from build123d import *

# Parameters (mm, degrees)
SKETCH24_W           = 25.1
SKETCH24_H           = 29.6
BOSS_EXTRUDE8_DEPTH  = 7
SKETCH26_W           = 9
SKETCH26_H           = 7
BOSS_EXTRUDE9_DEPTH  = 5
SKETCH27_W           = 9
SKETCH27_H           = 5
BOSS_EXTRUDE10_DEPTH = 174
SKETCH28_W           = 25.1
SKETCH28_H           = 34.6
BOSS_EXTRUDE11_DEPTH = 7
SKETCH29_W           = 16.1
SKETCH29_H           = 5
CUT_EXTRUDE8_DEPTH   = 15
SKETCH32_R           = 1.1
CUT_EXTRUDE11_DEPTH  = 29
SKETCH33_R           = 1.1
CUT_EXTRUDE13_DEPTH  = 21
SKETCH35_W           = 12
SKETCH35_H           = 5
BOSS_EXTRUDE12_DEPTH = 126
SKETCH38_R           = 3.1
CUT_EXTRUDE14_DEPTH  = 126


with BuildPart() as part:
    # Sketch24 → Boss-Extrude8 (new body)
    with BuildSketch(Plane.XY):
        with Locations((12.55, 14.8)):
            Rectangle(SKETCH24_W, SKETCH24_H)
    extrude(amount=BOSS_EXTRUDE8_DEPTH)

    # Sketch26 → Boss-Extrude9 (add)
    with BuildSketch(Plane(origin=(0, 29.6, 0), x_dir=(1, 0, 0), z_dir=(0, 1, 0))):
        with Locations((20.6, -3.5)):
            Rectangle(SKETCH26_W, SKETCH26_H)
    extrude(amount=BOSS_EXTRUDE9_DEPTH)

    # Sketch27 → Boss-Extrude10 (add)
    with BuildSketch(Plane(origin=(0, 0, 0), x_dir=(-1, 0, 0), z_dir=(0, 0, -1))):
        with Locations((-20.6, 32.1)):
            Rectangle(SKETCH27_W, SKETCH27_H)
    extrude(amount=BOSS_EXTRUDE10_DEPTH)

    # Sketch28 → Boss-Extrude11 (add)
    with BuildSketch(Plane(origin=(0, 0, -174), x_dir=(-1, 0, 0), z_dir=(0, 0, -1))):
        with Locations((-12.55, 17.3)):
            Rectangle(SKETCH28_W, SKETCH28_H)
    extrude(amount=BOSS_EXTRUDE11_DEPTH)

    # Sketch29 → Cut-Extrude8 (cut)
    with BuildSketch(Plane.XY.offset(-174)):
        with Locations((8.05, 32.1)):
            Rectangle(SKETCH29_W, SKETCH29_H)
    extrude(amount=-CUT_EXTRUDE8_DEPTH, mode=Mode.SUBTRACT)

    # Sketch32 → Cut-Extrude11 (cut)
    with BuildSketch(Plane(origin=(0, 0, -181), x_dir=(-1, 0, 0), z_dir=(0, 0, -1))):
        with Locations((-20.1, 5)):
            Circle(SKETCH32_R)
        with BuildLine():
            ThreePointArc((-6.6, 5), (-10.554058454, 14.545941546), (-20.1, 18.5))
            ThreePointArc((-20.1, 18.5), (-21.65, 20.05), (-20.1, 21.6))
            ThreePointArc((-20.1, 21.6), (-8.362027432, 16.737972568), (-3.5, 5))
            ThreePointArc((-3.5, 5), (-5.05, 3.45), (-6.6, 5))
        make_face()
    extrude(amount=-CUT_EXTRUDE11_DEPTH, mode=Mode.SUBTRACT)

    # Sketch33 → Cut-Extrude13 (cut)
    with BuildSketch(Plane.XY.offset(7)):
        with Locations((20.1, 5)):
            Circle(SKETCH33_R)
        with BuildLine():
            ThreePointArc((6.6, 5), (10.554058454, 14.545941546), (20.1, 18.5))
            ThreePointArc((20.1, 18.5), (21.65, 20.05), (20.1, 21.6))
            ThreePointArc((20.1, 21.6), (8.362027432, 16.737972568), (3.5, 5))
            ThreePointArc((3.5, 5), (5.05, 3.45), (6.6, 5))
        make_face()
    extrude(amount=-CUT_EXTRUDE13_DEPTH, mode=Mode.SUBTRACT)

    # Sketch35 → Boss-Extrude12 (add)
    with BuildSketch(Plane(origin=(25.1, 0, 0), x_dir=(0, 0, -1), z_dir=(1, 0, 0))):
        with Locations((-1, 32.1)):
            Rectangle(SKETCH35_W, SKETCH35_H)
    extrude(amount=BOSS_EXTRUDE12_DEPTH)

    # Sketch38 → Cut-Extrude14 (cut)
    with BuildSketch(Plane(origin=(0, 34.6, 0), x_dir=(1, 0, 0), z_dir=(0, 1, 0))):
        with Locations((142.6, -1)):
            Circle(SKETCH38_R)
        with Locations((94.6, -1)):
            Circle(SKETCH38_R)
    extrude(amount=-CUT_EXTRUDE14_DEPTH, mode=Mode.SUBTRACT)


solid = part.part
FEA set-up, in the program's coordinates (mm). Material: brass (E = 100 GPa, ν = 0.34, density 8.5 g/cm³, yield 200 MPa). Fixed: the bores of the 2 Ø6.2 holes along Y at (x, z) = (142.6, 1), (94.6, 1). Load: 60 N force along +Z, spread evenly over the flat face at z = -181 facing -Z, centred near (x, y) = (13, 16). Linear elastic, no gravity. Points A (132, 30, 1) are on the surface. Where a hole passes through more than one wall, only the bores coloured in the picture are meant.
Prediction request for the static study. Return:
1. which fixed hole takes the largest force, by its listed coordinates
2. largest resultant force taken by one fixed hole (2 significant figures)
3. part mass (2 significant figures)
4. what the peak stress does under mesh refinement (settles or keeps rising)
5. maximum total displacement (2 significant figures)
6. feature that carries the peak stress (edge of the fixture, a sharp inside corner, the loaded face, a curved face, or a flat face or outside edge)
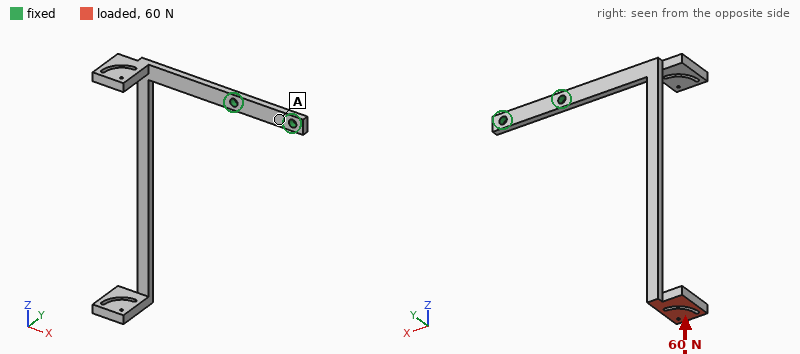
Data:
(94.6, 1)
72 N
210 g
keeps rising
2.8 mm
edge of the fixture
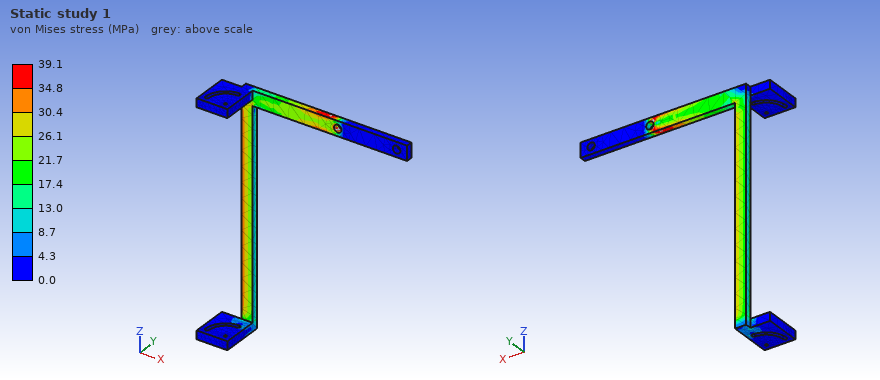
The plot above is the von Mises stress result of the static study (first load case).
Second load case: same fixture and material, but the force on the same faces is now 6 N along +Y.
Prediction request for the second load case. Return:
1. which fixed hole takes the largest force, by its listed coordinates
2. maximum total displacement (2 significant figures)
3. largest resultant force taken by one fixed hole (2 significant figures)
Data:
(94.6, 1)
2.3 mm
6.0 N
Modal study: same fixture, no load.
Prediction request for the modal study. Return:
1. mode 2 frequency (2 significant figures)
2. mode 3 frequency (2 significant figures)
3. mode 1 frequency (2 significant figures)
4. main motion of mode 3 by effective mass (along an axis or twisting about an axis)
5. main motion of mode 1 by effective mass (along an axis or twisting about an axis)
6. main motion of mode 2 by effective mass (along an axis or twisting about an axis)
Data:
66 Hz
160 Hz
34 Hz
along Y
along Y
along X
